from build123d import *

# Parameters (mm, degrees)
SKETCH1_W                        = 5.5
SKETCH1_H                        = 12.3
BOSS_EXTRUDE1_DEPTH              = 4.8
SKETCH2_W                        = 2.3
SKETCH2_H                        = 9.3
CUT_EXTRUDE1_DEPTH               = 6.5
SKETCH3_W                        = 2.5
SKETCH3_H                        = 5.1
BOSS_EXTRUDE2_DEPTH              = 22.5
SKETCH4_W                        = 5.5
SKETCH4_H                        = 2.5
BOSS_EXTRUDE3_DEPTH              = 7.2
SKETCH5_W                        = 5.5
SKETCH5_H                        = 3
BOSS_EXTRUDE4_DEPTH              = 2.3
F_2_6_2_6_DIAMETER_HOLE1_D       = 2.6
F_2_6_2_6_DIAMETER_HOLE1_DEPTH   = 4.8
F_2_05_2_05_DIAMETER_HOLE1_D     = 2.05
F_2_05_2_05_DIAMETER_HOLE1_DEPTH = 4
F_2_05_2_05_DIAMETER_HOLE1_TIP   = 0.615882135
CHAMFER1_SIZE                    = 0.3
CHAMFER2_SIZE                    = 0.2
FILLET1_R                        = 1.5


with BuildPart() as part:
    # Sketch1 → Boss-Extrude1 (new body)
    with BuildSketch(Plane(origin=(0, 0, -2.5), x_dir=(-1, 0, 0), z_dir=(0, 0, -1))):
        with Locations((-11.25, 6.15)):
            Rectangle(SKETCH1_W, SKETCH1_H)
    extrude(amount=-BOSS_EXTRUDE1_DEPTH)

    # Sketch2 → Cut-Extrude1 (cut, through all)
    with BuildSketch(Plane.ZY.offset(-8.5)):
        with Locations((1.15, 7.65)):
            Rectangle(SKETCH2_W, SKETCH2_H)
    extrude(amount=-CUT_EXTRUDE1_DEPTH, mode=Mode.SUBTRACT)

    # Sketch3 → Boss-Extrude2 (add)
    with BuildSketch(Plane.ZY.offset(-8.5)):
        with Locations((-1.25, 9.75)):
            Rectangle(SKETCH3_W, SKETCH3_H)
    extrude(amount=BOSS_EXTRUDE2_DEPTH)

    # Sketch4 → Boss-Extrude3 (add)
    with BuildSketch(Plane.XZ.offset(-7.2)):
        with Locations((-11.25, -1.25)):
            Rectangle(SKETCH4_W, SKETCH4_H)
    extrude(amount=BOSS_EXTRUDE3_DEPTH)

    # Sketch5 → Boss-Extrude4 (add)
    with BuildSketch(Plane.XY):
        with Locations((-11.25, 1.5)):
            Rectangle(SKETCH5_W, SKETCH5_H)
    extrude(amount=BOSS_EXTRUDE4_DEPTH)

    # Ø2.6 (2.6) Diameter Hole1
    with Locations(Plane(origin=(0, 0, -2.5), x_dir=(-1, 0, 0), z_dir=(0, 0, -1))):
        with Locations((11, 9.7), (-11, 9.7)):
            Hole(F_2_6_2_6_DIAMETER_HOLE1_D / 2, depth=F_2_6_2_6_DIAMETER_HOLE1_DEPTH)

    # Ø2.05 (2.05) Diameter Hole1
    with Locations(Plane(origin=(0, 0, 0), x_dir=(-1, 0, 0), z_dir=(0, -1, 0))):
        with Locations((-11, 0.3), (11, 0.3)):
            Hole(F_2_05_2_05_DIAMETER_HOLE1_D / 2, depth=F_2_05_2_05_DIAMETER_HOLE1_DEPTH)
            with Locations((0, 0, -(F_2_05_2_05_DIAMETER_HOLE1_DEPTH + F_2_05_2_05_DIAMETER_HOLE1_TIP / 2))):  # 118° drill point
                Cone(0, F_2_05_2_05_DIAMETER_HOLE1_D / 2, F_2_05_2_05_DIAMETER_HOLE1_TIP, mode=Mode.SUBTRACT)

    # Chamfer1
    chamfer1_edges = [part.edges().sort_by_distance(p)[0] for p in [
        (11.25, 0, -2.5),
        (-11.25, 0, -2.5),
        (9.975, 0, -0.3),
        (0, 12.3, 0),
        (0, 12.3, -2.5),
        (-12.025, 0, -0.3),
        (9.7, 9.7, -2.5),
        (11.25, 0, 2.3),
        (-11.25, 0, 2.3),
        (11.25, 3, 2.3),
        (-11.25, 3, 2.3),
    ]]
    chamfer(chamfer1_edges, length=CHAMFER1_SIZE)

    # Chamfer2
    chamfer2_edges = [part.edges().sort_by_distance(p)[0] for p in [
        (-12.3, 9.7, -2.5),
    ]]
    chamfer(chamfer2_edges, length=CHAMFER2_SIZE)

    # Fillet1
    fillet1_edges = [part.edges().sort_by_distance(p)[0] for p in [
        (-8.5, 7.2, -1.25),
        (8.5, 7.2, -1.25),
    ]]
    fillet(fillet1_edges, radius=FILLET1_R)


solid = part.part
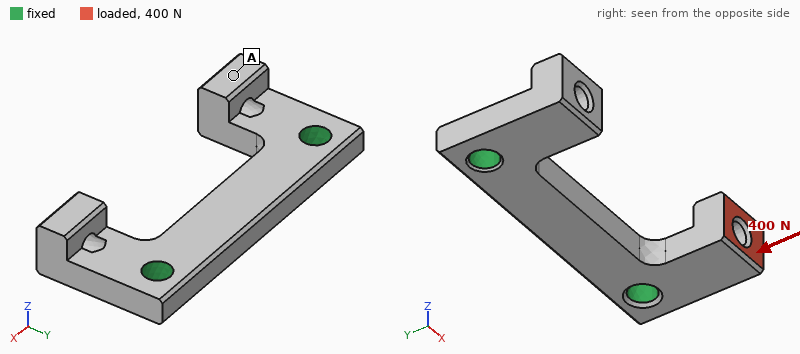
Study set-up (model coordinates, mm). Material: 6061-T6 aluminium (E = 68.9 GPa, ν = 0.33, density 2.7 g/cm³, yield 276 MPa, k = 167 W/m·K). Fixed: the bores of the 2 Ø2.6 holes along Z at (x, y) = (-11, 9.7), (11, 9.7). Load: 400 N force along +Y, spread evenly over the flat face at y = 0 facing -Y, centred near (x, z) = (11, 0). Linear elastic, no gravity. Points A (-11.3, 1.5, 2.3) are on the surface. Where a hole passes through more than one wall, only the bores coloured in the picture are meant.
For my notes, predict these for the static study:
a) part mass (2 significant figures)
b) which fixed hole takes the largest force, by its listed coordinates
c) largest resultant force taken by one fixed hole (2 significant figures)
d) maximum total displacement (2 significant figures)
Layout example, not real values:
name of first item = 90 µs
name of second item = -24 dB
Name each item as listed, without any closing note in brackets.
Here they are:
part mass = 1.6 g
which fixed hole takes the largest force, by its listed coordinates = (11, 9.7)
largest resultant force taken by one fixed hole = 400 N
maximum total displacement = 51 µm
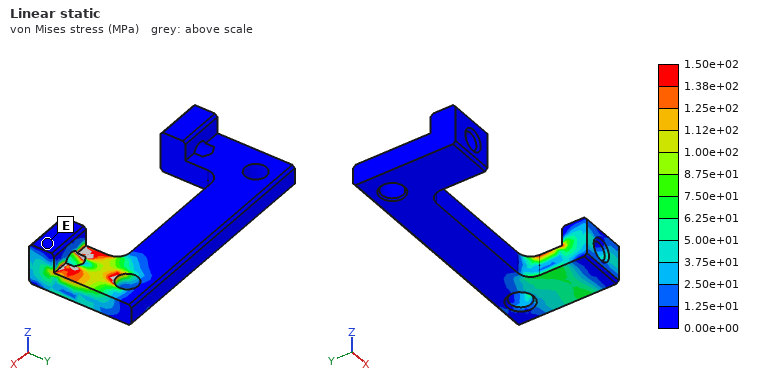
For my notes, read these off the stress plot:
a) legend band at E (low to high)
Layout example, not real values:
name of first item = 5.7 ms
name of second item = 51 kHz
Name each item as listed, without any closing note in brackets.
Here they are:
legend band at E = 0.00e+00 to 1.25e+01 MPa
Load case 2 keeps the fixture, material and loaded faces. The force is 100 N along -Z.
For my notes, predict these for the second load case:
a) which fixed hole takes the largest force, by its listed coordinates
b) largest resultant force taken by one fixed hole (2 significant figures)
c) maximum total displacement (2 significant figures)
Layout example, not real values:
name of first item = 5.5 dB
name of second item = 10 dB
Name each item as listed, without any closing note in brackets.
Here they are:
which fixed hole takes the largest force, by its listed coordinates = (11, 9.7)
largest resultant force taken by one fixed hole = 100 N
maximum total displacement = 58 µm
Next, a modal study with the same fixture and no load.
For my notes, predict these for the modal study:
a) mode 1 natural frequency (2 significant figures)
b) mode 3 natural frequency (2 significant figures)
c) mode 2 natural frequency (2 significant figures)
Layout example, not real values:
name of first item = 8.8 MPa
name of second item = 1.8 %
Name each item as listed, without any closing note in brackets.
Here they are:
mode 1 natural frequency = 19 kHz
mode 3 natural frequency = 28 kHz
mode 2 natural frequency = 19 kHz
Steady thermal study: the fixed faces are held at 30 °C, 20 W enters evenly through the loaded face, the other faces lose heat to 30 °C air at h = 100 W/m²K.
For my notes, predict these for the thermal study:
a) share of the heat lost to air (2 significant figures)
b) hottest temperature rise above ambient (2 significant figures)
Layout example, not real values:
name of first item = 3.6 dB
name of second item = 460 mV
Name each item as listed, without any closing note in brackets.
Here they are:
share of the heat lost to air = 4.7 %
hottest temperature rise above ambient = 78 K
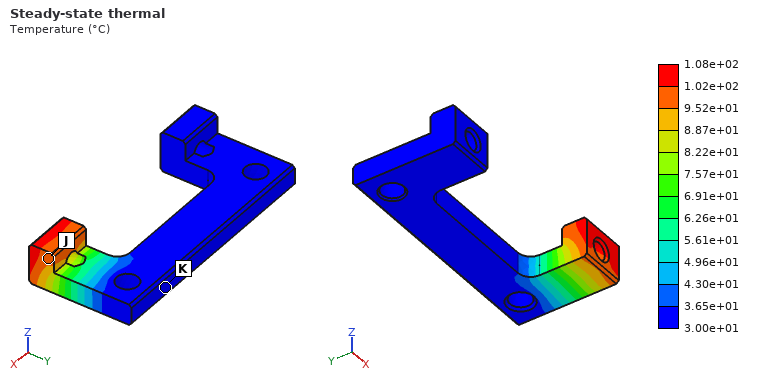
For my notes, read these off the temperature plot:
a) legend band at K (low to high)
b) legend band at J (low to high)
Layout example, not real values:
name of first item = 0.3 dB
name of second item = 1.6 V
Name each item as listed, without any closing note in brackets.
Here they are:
legend band at K = 3.00e+01 to 3.65e+01 °C
legend band at J = 9.52e+01 to 1.02e+02 °C
